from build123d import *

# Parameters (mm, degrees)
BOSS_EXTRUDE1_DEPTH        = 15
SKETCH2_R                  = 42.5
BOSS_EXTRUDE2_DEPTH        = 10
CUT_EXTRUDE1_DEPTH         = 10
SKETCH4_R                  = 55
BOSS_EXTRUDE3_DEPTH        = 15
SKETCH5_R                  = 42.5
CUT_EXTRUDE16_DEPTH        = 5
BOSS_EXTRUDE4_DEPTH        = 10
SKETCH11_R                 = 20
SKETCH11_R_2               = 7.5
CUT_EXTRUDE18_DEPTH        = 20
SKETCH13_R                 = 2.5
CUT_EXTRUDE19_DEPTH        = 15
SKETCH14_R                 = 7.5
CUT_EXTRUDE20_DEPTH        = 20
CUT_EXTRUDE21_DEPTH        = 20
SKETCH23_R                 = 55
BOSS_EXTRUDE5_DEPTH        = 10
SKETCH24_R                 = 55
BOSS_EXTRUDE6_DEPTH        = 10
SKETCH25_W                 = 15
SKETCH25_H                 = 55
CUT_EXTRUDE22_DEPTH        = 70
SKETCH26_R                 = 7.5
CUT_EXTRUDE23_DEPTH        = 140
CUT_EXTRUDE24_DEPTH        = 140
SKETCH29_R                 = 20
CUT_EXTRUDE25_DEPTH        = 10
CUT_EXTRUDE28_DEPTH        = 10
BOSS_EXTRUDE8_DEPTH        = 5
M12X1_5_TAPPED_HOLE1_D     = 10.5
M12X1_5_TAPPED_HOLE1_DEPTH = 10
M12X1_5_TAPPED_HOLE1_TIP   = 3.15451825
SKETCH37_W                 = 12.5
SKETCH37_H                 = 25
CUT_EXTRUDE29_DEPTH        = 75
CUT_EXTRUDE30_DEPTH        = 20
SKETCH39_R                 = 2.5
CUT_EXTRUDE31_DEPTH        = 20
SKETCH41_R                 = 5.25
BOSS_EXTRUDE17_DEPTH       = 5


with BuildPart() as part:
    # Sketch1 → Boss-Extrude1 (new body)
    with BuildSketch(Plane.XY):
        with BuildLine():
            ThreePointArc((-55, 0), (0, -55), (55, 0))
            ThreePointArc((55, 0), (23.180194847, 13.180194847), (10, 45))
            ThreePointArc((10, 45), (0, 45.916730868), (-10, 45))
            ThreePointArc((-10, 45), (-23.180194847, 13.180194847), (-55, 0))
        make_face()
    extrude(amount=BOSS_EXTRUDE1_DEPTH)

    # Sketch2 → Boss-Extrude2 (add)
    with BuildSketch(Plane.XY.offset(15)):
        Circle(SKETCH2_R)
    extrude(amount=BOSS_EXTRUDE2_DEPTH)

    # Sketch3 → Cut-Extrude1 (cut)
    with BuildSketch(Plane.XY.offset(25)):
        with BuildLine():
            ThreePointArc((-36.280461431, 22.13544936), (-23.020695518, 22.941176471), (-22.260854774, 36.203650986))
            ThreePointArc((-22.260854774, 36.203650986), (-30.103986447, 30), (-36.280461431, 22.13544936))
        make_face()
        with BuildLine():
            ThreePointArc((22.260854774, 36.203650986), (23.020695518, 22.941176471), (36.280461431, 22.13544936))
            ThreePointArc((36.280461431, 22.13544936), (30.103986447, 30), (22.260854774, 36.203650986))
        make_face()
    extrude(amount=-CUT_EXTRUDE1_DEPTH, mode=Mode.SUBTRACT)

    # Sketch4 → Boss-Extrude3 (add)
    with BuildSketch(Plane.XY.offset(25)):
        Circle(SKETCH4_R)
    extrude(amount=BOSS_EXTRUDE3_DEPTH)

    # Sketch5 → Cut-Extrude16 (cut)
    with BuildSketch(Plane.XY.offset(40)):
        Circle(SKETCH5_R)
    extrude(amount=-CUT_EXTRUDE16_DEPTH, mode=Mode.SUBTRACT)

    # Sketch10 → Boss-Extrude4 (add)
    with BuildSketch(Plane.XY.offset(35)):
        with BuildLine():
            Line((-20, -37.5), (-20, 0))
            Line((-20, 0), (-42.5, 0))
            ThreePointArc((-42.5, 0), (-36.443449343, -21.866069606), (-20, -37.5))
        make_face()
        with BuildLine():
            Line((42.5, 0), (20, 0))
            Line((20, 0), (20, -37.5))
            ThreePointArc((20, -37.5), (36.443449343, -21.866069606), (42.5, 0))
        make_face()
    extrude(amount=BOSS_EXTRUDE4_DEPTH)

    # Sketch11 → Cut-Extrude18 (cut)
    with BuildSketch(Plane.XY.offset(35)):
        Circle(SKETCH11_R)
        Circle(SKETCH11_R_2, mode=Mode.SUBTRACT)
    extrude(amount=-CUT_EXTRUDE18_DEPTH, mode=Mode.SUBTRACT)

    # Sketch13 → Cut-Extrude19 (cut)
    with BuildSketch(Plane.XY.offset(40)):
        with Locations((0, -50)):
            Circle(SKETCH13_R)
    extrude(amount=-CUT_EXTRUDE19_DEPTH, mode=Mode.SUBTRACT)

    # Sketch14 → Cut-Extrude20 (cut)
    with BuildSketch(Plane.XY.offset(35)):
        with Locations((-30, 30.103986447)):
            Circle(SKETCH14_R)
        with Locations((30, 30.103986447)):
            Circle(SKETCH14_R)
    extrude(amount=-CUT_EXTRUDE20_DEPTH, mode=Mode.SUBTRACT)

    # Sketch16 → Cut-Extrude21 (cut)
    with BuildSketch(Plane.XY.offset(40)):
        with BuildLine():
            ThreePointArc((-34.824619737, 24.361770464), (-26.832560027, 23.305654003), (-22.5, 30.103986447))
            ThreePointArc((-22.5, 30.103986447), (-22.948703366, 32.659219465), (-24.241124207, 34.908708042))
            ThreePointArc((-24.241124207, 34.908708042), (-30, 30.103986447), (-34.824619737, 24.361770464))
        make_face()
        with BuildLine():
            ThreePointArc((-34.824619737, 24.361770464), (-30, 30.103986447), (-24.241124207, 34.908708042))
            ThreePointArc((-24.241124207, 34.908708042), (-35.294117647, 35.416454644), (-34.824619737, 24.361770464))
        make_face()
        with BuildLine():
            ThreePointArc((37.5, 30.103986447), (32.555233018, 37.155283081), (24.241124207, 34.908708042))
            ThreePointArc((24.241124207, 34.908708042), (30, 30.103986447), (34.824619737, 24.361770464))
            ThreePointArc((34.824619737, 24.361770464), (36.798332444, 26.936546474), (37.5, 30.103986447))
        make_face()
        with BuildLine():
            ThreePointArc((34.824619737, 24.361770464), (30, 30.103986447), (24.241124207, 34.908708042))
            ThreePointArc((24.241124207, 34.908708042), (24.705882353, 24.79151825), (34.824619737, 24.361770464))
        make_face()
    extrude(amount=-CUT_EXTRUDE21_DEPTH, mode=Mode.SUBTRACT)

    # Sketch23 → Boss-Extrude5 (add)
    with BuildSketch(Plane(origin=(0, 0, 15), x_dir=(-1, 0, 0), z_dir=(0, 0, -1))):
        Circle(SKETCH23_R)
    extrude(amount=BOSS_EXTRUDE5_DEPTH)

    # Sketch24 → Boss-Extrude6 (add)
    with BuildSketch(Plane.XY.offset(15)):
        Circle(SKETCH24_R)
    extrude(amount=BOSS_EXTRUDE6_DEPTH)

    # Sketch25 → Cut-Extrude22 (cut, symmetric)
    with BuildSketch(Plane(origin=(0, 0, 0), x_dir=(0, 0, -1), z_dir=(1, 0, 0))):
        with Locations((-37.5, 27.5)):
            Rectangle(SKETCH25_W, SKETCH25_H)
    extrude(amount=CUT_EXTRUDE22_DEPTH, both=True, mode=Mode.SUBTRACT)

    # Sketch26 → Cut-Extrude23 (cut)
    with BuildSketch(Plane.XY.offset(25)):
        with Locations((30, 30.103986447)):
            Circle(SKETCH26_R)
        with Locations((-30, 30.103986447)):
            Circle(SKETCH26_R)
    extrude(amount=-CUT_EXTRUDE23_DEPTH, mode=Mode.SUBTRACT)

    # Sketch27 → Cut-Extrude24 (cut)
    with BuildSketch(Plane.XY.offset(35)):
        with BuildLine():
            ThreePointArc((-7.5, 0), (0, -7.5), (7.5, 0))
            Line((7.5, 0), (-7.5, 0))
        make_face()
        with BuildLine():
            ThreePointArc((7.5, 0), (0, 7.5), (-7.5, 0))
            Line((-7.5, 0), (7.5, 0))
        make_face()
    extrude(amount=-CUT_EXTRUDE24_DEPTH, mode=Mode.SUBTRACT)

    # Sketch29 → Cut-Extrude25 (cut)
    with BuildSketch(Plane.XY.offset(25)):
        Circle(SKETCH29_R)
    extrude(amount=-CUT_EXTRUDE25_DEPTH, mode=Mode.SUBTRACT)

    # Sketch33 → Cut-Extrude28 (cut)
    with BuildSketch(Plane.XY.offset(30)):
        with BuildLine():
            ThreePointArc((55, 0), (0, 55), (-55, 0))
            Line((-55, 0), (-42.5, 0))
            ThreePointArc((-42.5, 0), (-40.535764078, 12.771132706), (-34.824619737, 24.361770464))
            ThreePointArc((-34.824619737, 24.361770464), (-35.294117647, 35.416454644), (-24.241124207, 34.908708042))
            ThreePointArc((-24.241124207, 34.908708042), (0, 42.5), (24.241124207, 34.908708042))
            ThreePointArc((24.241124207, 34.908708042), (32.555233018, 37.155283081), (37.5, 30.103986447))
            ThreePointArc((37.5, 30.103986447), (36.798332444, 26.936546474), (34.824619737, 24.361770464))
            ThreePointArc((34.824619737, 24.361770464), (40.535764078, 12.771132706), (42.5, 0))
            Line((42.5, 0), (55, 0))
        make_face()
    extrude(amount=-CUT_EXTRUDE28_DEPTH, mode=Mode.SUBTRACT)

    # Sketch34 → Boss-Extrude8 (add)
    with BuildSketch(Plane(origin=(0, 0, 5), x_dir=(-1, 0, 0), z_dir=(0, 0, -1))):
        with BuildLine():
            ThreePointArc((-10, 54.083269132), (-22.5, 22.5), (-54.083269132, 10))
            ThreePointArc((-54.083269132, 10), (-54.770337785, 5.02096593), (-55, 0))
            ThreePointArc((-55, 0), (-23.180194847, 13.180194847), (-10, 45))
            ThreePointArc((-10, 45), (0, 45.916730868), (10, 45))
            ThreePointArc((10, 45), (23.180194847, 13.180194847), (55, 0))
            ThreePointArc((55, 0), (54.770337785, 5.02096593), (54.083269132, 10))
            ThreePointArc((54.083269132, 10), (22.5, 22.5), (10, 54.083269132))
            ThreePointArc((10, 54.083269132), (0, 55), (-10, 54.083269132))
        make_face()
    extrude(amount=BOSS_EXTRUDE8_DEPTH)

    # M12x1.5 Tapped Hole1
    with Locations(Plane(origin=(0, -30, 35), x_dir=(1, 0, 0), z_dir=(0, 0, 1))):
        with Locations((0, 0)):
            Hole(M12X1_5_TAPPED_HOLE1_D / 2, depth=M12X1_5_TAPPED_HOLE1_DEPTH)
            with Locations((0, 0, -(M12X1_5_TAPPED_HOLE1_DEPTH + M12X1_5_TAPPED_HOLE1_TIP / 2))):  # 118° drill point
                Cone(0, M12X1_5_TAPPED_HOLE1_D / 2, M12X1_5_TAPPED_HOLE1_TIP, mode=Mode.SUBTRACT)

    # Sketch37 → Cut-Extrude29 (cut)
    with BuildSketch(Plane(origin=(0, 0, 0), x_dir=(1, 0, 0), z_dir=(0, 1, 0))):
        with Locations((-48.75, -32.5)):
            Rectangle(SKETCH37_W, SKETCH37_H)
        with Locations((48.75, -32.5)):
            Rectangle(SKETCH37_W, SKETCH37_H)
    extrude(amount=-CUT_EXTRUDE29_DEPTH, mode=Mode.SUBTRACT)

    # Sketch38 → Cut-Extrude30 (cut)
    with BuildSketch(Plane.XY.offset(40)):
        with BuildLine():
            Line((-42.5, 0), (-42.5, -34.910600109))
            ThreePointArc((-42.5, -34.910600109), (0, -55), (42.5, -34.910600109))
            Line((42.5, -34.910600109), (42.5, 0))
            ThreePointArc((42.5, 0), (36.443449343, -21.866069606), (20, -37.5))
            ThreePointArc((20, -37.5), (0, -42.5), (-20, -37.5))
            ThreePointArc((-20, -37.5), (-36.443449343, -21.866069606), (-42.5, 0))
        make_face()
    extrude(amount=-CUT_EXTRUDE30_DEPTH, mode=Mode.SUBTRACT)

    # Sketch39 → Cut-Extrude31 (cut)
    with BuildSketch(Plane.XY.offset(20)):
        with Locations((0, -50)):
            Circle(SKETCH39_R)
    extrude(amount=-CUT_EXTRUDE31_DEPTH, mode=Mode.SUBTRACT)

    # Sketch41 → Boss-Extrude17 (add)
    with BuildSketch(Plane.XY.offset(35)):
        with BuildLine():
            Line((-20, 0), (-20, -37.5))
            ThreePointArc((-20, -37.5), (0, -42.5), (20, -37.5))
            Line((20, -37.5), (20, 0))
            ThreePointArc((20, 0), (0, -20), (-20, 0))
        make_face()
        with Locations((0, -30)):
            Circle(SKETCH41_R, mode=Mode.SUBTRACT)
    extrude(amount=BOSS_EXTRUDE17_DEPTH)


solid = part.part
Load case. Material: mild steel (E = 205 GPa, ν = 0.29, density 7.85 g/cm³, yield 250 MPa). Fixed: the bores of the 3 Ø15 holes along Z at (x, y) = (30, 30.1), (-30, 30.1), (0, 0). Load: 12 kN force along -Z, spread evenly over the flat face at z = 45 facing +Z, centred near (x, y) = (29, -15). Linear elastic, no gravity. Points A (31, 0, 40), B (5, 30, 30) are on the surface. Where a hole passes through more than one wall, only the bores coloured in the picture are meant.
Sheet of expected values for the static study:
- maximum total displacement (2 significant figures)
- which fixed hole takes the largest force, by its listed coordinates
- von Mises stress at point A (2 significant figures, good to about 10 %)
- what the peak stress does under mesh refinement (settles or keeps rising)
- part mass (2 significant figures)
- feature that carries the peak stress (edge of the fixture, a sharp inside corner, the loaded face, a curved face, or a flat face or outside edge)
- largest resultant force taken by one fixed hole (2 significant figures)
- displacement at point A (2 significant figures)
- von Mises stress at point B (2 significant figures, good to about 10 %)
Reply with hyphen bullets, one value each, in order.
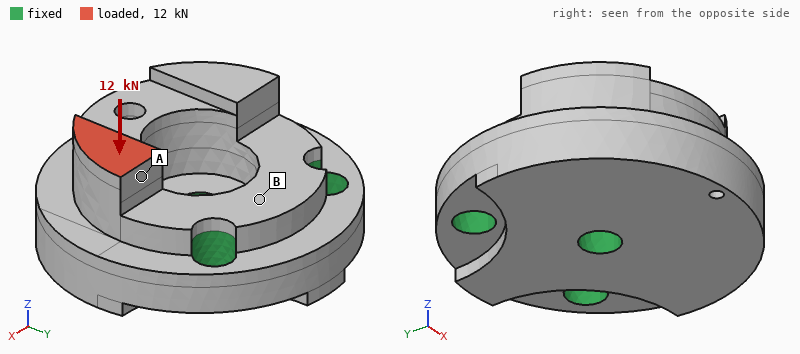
- 21 µm
- (0, 0)
- 22 MPa
- keeps rising
- 1.8 kg
- edge of the fixture
- 11 kN
- 13 µm
- 9.3 MPa
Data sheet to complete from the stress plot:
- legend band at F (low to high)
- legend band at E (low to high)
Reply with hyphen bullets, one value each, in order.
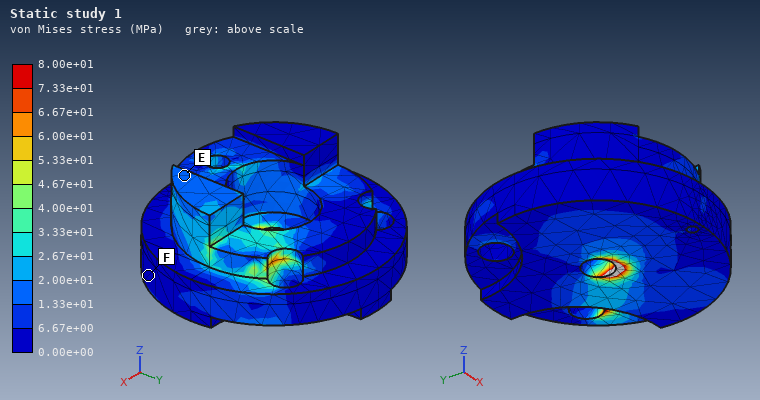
- 0.00e+00 to 6.67e+00 MPa
- 1.33e+01 to 2.00e+01 MPa
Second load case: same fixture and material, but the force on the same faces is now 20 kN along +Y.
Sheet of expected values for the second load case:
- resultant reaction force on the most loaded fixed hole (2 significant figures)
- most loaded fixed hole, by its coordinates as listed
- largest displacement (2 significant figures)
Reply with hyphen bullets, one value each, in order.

- 20 kN
- (30, 30.1)
- 51 µm
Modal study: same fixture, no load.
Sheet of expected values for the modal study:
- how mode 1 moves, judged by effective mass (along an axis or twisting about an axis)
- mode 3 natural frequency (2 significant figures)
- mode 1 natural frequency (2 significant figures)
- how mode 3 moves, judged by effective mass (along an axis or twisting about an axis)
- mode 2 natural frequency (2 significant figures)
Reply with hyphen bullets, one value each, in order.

- along Z
- 9500 Hz
- 5000 Hz
- along X
- 6000 Hz
